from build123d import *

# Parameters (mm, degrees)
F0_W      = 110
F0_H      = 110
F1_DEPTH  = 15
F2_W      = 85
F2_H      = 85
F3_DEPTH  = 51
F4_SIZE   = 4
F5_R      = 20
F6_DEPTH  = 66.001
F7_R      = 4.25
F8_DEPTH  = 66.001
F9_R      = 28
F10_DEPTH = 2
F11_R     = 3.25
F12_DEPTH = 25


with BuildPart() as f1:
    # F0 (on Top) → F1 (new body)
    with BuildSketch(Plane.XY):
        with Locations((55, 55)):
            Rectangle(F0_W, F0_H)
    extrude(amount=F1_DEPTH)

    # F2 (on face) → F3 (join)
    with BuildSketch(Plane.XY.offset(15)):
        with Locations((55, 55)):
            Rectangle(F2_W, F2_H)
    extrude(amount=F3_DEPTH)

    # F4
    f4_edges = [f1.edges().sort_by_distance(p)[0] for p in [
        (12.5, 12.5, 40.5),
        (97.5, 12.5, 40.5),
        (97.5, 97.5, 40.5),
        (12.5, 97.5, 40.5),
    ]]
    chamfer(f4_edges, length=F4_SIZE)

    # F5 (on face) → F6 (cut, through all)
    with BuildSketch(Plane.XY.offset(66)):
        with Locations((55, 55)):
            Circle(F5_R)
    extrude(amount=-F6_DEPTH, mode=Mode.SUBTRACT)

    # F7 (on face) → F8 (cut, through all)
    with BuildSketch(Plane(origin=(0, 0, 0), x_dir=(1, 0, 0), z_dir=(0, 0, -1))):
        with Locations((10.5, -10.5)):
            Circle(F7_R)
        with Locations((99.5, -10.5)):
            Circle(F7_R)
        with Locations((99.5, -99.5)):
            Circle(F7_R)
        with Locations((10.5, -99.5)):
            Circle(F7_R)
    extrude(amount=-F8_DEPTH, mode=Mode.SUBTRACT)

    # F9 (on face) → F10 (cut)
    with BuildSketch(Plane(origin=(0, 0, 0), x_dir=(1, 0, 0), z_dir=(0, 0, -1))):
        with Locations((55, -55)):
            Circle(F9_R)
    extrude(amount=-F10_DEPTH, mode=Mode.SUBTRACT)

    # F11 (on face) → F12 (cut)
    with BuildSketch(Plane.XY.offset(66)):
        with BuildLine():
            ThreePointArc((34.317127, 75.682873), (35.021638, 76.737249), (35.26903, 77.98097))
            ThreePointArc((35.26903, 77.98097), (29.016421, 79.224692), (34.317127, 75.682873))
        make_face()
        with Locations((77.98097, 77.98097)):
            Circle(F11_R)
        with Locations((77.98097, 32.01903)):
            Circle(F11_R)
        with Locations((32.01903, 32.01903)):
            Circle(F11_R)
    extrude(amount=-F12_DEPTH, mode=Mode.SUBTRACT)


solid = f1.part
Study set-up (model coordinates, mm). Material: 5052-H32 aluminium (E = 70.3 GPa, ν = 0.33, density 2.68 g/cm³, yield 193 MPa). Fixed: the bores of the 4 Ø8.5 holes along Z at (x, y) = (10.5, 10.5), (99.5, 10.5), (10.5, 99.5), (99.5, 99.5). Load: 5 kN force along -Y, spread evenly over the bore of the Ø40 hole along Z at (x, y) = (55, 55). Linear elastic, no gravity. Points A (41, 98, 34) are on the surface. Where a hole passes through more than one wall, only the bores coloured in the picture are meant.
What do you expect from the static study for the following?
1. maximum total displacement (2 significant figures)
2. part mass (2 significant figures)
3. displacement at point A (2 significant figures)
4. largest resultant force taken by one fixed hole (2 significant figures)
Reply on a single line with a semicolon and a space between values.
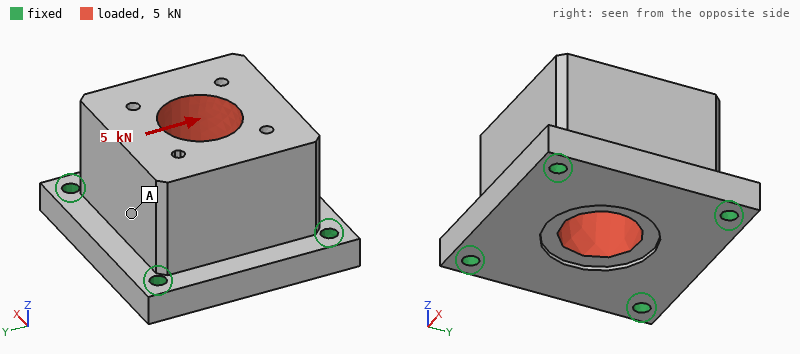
4.5 µm; 1.2 kg; 3.0 µm; 1.6 kN
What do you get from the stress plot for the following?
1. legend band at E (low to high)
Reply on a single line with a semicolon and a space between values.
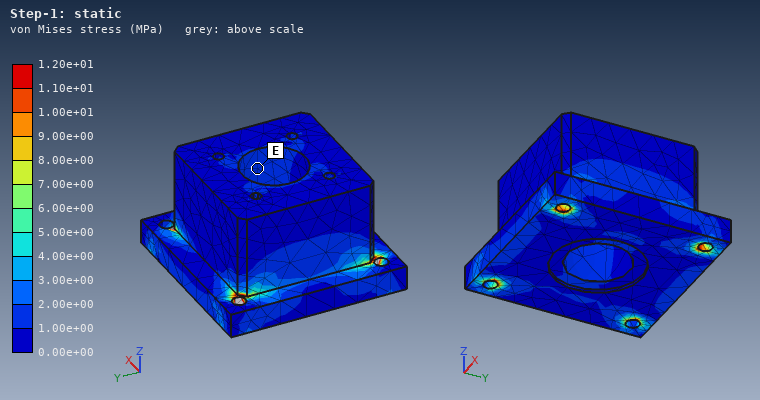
1.00e+00 to 2.00e+00 MPa
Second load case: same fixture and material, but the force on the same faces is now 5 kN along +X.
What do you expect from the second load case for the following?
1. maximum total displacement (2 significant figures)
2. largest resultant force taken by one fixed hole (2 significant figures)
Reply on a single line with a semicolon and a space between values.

4.5 µm; 1.6 kN
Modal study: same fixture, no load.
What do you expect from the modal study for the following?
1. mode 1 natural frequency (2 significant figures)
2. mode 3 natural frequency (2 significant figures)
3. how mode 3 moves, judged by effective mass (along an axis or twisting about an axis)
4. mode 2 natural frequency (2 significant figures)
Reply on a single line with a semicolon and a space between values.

6000 Hz; 6400 Hz; along Z; 6000 Hz
